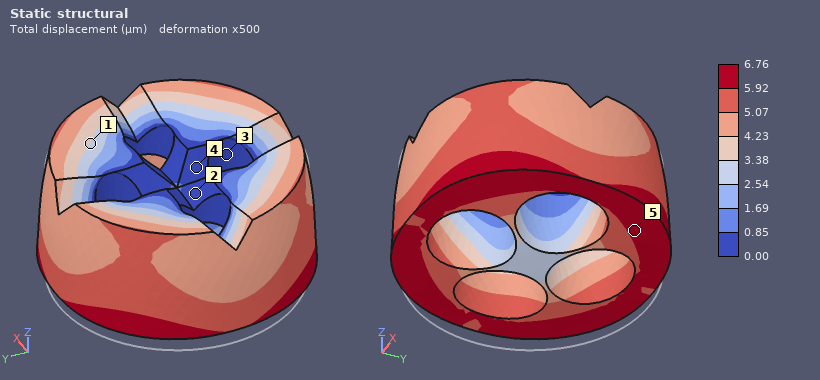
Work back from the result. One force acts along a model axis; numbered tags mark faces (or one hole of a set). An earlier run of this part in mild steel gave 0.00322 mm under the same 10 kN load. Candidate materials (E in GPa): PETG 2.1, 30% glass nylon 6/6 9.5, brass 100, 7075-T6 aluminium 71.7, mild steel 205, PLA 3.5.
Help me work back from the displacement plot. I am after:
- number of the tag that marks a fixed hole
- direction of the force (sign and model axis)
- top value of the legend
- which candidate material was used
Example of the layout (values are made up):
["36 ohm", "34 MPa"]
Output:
["3", "+Z", "6.76 µm", "brass"]
